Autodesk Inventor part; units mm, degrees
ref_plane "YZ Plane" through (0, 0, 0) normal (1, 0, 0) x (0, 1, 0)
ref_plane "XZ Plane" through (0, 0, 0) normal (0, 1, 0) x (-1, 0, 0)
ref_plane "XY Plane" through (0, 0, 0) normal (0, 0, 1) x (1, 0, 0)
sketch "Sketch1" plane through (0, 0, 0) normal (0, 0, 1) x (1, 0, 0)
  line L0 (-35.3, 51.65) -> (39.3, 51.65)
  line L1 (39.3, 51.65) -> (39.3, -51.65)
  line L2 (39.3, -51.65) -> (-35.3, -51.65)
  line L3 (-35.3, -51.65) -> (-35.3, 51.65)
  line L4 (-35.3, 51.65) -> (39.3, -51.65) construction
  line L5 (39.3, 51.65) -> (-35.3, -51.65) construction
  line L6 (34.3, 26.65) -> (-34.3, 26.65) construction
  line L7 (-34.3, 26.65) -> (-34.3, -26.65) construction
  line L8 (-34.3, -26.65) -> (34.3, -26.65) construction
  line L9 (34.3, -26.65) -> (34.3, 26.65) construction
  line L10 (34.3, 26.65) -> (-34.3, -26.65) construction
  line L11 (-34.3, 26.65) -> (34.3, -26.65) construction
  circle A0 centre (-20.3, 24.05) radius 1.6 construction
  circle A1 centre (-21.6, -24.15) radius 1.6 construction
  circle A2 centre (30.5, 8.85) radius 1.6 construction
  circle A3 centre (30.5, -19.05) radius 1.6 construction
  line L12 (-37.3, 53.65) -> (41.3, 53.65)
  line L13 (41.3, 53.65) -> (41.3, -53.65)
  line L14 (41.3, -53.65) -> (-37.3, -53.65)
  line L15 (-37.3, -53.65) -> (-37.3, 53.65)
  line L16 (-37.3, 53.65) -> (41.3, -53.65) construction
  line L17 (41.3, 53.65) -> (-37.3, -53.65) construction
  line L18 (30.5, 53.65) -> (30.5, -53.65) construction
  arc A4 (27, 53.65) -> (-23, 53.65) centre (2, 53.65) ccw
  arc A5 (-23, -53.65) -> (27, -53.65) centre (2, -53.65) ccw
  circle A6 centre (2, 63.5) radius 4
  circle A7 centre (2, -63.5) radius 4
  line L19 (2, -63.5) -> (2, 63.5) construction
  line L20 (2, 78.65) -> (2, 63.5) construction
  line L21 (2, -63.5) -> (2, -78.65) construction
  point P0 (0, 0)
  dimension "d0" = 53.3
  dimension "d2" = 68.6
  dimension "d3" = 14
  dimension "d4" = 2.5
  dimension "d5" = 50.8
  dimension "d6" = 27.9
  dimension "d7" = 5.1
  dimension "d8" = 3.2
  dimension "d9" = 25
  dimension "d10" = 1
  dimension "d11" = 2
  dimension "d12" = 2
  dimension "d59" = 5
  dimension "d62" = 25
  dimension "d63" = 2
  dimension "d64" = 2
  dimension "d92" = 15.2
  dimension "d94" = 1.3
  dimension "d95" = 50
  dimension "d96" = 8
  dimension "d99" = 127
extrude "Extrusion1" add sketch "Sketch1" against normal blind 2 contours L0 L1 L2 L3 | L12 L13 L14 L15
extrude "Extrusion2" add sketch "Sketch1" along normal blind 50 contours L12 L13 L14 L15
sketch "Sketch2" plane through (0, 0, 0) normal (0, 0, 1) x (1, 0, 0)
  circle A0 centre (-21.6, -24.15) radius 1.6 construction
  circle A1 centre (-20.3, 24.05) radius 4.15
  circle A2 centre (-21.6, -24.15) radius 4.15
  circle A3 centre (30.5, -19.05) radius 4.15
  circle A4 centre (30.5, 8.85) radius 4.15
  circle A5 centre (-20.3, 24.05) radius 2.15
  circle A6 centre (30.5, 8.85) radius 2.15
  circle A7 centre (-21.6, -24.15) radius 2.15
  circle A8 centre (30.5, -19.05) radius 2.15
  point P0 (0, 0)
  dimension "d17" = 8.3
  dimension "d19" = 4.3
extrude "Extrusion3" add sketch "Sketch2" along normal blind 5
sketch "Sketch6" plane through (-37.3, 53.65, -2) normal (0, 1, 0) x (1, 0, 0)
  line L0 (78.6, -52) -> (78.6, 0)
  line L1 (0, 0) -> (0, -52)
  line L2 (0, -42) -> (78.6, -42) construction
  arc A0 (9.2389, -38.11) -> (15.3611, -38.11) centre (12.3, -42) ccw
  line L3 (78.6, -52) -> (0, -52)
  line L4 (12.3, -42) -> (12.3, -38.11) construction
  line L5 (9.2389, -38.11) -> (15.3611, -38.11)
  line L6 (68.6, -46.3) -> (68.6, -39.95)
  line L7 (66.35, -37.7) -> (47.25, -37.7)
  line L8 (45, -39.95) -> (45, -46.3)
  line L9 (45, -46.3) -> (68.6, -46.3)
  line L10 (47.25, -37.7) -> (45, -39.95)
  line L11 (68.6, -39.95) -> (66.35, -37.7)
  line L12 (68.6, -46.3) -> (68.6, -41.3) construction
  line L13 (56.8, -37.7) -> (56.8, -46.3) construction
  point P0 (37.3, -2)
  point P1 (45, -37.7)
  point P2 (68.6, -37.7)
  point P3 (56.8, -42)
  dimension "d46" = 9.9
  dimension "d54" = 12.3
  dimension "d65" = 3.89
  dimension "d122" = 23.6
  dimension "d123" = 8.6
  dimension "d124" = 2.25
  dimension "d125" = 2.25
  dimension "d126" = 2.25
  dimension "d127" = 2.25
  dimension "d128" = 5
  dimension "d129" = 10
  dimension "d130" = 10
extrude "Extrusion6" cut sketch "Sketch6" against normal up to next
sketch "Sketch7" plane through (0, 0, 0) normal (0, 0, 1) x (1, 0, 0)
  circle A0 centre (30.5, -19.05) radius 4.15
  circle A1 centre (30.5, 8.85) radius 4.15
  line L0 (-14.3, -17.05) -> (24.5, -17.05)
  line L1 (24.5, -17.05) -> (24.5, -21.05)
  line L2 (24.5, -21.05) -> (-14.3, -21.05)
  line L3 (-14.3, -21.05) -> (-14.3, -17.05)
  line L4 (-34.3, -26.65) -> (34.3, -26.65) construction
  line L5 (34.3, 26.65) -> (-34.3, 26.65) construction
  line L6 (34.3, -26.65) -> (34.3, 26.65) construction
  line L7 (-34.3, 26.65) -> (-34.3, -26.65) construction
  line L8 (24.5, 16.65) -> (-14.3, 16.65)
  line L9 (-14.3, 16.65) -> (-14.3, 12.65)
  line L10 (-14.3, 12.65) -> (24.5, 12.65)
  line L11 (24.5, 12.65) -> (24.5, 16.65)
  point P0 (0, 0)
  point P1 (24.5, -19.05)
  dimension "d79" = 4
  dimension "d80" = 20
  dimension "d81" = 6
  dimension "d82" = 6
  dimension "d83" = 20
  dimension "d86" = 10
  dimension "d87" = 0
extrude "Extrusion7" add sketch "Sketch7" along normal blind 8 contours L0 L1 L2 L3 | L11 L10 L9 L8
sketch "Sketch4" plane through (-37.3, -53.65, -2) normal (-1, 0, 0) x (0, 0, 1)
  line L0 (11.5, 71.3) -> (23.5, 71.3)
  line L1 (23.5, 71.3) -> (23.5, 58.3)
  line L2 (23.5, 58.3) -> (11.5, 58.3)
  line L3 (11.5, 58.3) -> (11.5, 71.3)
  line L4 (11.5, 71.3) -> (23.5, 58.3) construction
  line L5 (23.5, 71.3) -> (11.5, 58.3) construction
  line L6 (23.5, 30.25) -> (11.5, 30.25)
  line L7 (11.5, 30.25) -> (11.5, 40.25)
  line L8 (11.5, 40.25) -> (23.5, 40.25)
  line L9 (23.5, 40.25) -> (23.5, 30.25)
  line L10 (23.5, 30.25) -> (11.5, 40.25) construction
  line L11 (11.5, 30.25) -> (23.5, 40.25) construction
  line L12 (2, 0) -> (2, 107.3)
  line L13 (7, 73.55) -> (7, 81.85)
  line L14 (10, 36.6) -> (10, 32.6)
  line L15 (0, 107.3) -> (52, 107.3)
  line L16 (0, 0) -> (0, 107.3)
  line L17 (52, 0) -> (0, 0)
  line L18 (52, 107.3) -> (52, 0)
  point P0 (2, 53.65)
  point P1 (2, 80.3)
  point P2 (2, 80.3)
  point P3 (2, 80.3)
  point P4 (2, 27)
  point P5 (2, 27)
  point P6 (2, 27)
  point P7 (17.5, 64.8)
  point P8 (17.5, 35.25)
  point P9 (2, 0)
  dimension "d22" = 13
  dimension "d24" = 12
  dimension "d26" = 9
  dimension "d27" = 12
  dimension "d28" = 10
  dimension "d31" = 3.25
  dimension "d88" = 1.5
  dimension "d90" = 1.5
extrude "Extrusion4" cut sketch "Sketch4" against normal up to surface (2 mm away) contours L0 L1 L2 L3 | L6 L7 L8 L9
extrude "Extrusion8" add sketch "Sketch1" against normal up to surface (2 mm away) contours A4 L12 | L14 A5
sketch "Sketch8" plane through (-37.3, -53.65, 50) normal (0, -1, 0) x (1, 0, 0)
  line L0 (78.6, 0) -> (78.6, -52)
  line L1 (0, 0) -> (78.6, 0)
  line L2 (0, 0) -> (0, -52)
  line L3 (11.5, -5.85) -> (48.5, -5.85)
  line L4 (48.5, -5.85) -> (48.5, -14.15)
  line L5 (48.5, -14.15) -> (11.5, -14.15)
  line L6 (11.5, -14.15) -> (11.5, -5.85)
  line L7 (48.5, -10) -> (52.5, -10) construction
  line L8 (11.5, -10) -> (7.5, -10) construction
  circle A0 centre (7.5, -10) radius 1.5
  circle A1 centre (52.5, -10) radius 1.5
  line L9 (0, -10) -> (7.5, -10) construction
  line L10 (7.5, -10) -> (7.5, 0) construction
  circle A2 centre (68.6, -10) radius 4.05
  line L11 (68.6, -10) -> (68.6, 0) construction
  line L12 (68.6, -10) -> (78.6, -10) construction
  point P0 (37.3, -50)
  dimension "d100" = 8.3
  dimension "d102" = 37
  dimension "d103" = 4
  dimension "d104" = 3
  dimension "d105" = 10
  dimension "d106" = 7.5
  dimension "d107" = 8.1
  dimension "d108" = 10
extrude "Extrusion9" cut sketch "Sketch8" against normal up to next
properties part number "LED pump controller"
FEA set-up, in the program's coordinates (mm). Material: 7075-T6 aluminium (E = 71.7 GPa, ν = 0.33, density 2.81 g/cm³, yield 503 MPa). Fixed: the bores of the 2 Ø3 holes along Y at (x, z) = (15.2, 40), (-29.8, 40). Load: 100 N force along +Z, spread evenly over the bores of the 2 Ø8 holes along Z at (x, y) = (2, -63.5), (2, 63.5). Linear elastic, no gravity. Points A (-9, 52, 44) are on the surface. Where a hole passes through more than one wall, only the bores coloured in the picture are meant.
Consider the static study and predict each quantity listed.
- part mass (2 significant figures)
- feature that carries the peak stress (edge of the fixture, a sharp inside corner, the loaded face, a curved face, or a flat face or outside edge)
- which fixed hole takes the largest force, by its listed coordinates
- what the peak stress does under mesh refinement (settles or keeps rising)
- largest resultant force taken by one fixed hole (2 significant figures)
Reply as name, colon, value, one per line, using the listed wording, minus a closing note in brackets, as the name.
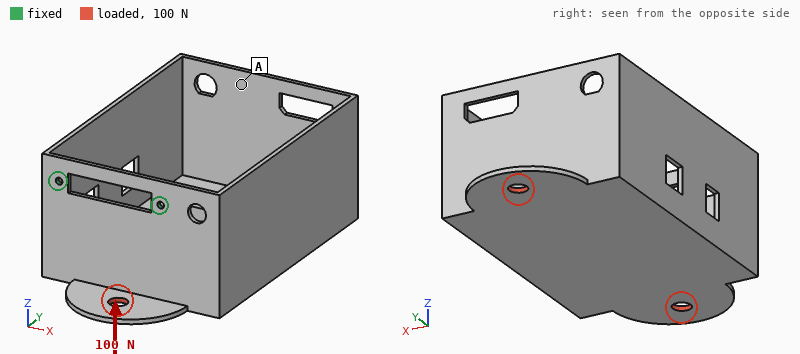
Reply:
part mass: 160 g
feature that carries the peak stress: edge of the fixture
which fixed hole takes the largest force, by its listed coordinates: (15.2, 40)
what the peak stress does under mesh refinement: keeps rising
largest resultant force taken by one fixed hole: 75 N
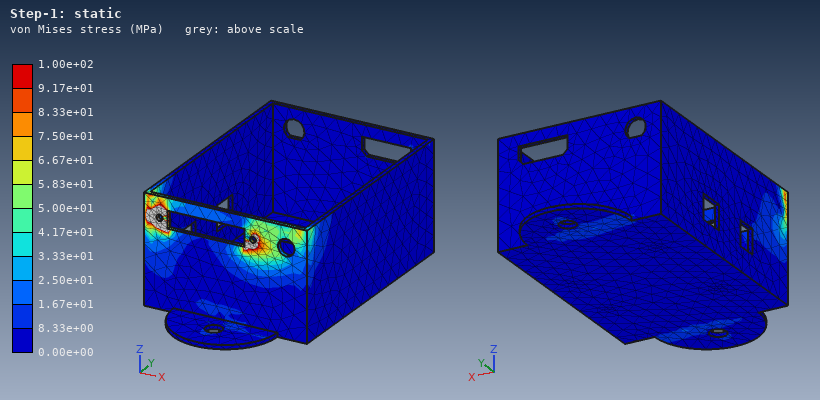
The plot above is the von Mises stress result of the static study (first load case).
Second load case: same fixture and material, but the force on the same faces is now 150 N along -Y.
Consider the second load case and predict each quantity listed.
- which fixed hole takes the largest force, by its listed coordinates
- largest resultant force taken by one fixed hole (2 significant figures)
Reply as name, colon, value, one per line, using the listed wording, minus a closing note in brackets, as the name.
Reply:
which fixed hole takes the largest force, by its listed coordinates: (15.2, 40)
largest resultant force taken by one fixed hole: 91 N
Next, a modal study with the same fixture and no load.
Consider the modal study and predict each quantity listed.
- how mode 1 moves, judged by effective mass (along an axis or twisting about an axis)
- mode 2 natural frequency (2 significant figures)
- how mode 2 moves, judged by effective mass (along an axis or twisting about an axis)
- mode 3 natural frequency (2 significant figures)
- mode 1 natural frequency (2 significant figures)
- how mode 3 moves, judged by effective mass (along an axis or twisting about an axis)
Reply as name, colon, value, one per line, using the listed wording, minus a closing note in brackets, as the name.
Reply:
how mode 1 moves, judged by effective mass: along Z
mode 2 natural frequency: 150 Hz
how mode 2 moves, judged by effective mass: along X
mode 3 natural frequency: 470 Hz
mode 1 natural frequency: 110 Hz
how mode 3 moves, judged by effective mass: along Y
